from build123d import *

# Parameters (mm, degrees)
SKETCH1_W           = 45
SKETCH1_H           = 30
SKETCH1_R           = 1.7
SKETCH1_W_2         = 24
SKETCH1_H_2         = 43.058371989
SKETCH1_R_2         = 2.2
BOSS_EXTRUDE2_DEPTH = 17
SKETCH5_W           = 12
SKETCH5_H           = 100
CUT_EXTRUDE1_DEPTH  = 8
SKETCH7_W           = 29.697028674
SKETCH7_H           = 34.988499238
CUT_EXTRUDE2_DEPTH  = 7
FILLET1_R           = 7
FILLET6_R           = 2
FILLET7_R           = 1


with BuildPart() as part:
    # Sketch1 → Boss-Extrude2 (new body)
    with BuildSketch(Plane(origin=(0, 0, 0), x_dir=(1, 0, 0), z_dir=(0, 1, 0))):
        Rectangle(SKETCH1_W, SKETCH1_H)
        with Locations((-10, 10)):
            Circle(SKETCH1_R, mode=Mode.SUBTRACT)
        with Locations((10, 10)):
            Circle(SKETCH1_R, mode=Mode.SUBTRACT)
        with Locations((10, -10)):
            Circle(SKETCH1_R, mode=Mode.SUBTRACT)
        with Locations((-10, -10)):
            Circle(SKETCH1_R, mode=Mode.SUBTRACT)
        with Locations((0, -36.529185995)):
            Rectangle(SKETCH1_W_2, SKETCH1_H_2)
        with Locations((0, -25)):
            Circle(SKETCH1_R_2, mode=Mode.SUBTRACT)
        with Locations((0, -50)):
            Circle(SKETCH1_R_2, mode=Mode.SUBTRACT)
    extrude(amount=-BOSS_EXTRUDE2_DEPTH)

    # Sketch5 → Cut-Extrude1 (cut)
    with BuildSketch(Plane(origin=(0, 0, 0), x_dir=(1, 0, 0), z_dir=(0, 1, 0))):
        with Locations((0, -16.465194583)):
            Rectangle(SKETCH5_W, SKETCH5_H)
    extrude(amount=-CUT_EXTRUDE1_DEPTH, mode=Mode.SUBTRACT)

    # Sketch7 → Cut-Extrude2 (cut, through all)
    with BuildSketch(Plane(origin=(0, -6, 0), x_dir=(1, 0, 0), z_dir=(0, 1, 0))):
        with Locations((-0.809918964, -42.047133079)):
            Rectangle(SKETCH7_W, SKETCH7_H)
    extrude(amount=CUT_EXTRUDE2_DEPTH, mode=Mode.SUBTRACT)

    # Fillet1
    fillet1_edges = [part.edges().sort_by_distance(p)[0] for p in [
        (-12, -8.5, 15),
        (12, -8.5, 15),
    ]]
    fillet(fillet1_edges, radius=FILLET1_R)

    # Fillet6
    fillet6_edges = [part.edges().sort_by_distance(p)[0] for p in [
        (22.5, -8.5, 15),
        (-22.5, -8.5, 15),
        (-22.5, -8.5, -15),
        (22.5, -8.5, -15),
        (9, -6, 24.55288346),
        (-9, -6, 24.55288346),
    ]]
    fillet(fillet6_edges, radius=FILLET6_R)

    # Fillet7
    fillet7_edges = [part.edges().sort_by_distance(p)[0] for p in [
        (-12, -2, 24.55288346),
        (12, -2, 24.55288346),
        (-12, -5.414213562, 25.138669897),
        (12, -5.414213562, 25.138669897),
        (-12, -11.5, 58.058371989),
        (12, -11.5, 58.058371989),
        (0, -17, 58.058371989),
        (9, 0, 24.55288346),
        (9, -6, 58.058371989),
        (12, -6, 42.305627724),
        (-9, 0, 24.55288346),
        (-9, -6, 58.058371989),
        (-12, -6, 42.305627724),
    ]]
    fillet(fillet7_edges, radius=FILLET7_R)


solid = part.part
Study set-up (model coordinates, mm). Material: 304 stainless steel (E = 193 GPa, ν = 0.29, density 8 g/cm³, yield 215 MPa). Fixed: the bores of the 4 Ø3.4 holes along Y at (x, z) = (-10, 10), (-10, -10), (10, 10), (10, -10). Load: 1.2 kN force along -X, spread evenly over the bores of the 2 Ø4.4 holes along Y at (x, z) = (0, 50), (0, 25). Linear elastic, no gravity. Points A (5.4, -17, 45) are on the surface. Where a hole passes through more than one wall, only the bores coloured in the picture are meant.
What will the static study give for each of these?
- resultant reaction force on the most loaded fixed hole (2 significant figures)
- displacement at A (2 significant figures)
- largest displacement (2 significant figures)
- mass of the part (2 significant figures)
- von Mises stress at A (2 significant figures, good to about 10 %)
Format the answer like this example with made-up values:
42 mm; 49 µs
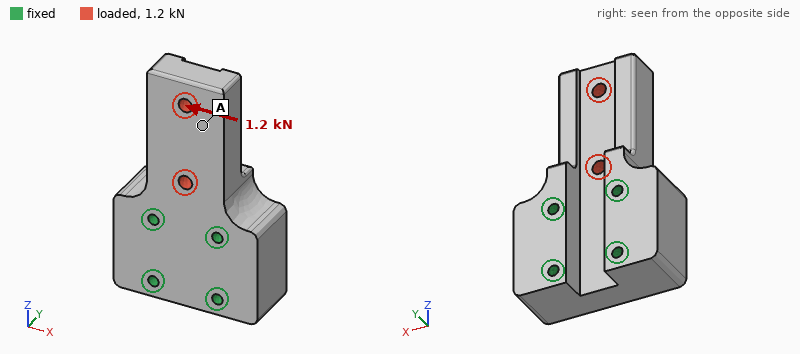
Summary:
1.4 kN; 4.8 µm; 7.9 µm; 240 g; 4.8 MPa
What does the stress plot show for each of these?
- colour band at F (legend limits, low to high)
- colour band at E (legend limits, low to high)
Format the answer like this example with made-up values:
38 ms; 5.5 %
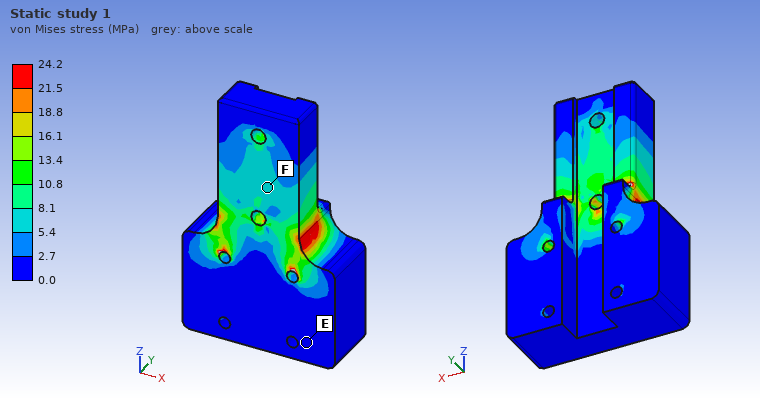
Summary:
5.4 to 8.1 MPa; 0.0 to 2.7 MPa
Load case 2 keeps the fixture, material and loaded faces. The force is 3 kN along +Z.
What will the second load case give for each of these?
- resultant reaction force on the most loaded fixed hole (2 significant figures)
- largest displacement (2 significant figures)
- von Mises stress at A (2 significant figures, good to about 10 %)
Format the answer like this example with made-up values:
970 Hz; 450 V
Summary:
1.3 kN; 5.4 µm; 9.6 MPa
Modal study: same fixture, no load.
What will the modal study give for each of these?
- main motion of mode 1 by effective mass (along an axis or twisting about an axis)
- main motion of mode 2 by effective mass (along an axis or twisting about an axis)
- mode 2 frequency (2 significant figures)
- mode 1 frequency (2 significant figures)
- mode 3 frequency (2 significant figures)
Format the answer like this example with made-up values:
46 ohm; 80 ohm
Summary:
along Y; along X; 8500 Hz; 4700 Hz; 12 kHz
